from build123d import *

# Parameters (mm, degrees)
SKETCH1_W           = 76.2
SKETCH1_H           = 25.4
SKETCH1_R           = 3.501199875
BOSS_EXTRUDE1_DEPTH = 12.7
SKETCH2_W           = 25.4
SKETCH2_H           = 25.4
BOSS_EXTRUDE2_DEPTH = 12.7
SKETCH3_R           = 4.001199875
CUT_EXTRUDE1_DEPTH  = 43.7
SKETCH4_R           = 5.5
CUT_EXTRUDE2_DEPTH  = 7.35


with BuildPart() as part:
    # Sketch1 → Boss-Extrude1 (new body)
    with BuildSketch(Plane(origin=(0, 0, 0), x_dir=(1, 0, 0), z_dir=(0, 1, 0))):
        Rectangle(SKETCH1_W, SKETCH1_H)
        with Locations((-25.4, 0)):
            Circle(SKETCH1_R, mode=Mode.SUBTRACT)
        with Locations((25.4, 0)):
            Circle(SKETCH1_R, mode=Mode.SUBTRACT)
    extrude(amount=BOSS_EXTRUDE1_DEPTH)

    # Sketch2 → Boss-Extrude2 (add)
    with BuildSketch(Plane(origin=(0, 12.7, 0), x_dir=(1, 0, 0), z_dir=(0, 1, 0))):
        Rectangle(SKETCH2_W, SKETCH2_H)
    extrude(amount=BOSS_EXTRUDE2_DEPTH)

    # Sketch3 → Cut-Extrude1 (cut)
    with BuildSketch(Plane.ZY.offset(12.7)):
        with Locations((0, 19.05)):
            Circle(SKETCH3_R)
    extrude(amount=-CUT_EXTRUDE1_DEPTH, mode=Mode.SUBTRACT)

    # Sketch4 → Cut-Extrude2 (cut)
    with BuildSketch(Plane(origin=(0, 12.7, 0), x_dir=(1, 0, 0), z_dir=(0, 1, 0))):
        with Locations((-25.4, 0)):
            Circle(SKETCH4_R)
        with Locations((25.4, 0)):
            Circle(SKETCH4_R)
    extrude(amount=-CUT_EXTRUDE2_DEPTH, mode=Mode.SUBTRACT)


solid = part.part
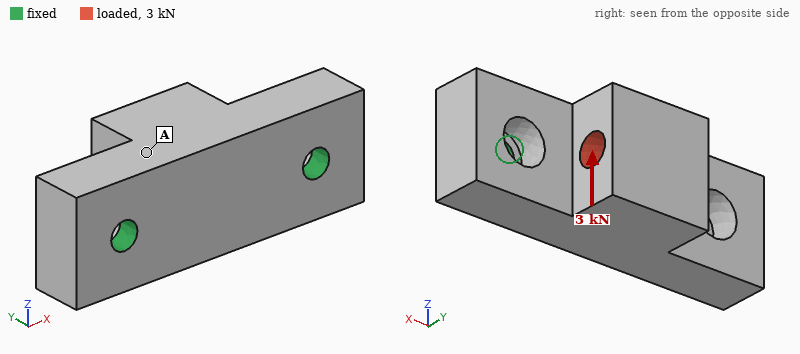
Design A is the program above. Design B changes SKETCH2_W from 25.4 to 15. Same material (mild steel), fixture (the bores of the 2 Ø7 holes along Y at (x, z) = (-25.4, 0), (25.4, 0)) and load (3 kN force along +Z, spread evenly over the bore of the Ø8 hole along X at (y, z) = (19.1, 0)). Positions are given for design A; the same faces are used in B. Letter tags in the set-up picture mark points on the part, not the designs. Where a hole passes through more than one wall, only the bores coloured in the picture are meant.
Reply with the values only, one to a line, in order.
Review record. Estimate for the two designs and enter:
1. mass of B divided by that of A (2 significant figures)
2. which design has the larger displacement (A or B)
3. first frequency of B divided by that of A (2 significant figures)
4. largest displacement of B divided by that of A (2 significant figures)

0.90
B
1.1
1.2
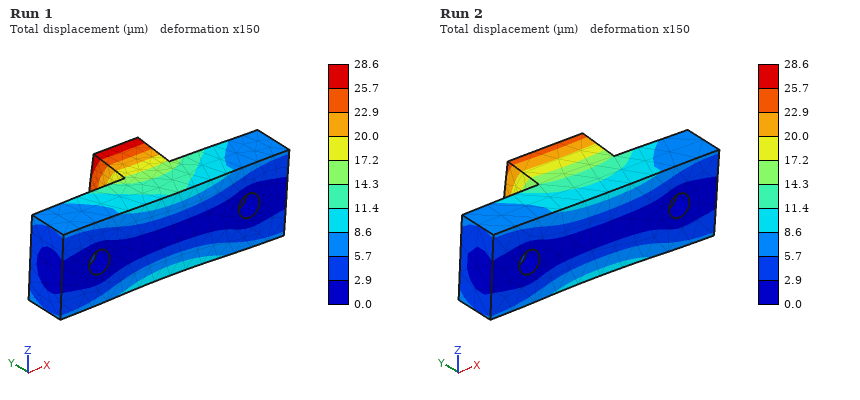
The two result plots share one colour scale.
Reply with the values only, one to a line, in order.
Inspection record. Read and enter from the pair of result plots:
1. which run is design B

Run 1
